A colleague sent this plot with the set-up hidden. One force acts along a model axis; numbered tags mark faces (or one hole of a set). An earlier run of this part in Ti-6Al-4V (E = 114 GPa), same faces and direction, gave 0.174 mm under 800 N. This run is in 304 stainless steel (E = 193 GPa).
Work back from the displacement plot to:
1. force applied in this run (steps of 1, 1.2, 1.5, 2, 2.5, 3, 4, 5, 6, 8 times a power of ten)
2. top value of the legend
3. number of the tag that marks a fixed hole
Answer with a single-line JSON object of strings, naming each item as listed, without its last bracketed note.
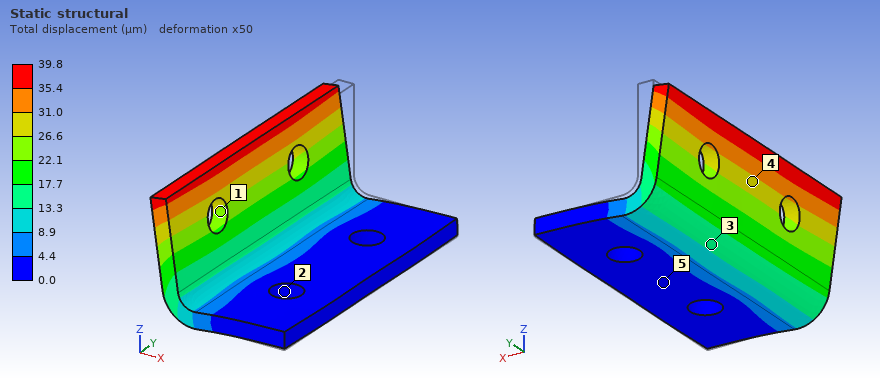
{"force applied in this run": "300 N", "top value of the legend": "39.8 µm", "number of the tag that marks a fixed hole": "2"}
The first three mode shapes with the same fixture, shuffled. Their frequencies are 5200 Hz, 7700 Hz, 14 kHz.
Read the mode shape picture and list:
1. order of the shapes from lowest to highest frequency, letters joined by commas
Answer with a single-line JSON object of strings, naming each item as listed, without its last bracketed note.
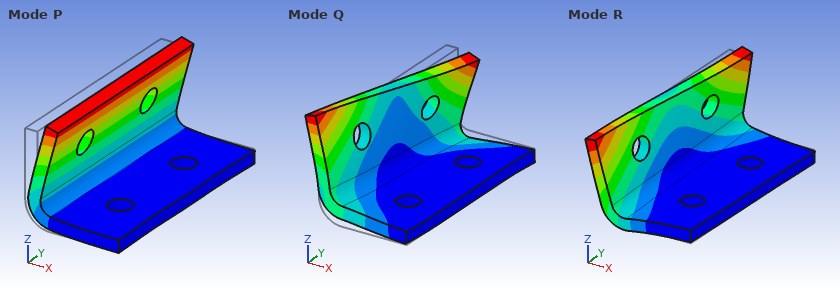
{"order of the shapes from lowest to highest frequency, letters joined by commas": "P, R, Q"}
